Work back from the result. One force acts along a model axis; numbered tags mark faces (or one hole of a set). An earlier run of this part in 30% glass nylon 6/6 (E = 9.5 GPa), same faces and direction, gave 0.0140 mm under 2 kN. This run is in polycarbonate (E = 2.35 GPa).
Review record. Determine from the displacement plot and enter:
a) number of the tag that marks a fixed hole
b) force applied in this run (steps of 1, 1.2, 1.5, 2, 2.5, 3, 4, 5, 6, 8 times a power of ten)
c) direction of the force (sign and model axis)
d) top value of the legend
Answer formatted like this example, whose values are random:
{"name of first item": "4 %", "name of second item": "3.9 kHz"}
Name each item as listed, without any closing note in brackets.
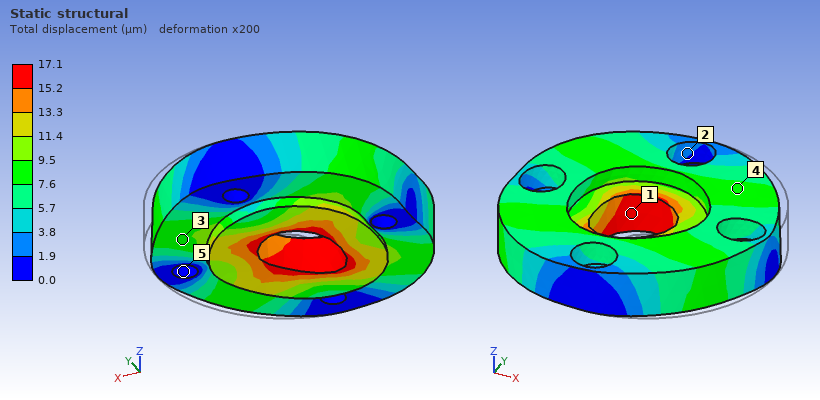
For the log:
{"number of the tag that marks a fixed hole": "5", "force applied in this run": "600 N", "direction of the force": "-X", "top value of the legend": "17.1 µm"}
